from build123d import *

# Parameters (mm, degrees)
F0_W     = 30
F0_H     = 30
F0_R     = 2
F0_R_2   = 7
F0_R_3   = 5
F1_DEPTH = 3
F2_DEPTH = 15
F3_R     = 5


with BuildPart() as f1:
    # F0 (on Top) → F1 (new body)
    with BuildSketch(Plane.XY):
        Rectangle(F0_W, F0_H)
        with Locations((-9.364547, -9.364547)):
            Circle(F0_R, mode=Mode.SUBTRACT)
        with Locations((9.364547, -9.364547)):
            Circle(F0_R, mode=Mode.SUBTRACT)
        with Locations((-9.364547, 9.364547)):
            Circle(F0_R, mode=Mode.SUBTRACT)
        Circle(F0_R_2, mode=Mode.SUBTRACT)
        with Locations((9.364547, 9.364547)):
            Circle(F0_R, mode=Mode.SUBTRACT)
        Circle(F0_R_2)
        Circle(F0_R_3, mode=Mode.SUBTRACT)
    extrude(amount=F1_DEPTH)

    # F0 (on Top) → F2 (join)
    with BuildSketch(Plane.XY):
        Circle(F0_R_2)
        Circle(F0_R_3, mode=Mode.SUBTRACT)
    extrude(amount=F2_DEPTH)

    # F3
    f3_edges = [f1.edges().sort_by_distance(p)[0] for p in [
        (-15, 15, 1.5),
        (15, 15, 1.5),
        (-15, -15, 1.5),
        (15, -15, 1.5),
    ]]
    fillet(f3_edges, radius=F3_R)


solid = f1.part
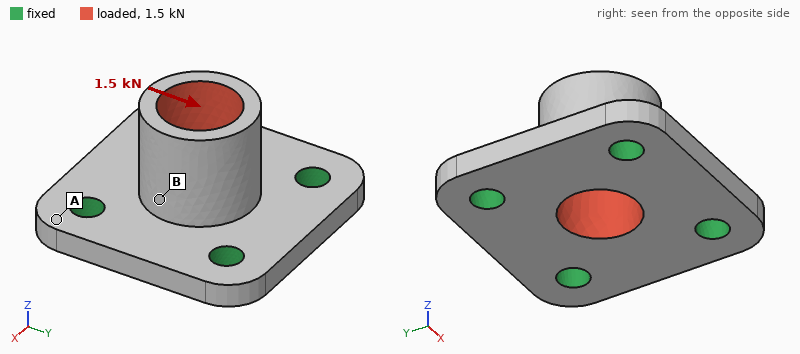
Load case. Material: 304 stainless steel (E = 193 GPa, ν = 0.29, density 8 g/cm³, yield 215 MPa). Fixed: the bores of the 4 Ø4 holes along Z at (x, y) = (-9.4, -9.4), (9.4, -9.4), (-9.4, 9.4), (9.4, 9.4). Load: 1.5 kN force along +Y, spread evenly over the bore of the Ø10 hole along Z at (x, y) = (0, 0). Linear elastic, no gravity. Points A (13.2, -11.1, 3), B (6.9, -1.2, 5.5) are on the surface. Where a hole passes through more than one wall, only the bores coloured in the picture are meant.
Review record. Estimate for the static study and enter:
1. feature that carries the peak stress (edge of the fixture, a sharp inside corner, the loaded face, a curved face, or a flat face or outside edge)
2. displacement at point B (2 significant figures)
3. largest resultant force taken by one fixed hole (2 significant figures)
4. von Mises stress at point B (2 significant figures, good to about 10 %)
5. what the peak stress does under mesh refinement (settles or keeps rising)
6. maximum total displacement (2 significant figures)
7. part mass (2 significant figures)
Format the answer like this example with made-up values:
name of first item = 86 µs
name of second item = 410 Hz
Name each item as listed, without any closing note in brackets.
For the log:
feature that carries the peak stress = edge of the fixture
displacement at point B = 2.9 µm
largest resultant force taken by one fixed hole = 500 N
von Mises stress at point B = 25 MPa
what the peak stress does under mesh refinement = keeps rising
maximum total displacement = 10 µm
part mass = 25 g
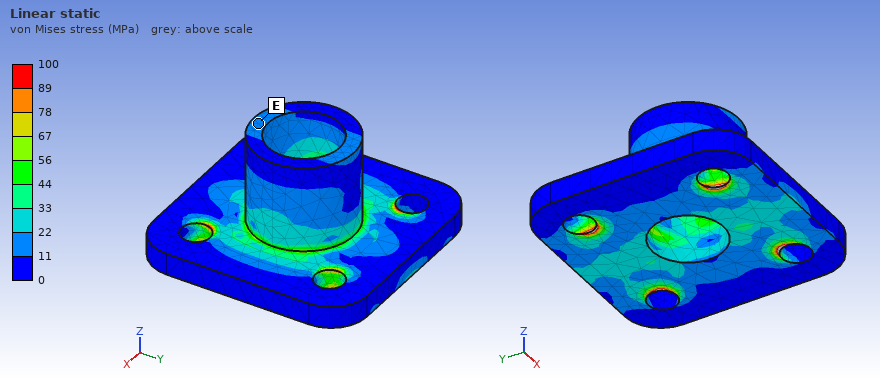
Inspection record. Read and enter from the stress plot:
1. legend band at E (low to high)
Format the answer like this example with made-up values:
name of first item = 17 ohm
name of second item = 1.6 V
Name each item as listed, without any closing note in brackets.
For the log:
legend band at E = 11 to 22 MPa
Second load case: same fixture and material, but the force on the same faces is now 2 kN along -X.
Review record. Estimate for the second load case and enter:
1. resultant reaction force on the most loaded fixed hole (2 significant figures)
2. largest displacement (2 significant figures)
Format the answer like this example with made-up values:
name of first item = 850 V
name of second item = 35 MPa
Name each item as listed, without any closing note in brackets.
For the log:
resultant reaction force on the most loaded fixed hole = 660 N
largest displacement = 14 µm
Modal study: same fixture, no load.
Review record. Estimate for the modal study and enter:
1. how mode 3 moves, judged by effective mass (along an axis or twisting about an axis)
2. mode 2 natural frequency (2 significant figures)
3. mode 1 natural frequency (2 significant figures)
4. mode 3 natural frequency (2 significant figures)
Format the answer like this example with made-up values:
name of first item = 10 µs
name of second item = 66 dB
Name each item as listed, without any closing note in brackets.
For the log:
how mode 3 moves, judged by effective mass = along Z
mode 2 natural frequency = 23 kHz
mode 1 natural frequency = 23 kHz
mode 3 natural frequency = 30 kHz
